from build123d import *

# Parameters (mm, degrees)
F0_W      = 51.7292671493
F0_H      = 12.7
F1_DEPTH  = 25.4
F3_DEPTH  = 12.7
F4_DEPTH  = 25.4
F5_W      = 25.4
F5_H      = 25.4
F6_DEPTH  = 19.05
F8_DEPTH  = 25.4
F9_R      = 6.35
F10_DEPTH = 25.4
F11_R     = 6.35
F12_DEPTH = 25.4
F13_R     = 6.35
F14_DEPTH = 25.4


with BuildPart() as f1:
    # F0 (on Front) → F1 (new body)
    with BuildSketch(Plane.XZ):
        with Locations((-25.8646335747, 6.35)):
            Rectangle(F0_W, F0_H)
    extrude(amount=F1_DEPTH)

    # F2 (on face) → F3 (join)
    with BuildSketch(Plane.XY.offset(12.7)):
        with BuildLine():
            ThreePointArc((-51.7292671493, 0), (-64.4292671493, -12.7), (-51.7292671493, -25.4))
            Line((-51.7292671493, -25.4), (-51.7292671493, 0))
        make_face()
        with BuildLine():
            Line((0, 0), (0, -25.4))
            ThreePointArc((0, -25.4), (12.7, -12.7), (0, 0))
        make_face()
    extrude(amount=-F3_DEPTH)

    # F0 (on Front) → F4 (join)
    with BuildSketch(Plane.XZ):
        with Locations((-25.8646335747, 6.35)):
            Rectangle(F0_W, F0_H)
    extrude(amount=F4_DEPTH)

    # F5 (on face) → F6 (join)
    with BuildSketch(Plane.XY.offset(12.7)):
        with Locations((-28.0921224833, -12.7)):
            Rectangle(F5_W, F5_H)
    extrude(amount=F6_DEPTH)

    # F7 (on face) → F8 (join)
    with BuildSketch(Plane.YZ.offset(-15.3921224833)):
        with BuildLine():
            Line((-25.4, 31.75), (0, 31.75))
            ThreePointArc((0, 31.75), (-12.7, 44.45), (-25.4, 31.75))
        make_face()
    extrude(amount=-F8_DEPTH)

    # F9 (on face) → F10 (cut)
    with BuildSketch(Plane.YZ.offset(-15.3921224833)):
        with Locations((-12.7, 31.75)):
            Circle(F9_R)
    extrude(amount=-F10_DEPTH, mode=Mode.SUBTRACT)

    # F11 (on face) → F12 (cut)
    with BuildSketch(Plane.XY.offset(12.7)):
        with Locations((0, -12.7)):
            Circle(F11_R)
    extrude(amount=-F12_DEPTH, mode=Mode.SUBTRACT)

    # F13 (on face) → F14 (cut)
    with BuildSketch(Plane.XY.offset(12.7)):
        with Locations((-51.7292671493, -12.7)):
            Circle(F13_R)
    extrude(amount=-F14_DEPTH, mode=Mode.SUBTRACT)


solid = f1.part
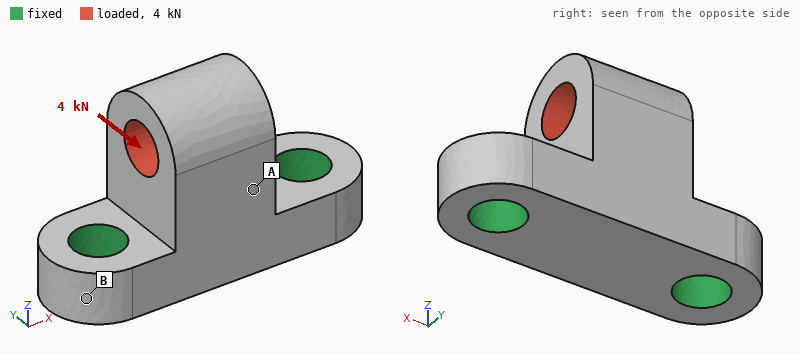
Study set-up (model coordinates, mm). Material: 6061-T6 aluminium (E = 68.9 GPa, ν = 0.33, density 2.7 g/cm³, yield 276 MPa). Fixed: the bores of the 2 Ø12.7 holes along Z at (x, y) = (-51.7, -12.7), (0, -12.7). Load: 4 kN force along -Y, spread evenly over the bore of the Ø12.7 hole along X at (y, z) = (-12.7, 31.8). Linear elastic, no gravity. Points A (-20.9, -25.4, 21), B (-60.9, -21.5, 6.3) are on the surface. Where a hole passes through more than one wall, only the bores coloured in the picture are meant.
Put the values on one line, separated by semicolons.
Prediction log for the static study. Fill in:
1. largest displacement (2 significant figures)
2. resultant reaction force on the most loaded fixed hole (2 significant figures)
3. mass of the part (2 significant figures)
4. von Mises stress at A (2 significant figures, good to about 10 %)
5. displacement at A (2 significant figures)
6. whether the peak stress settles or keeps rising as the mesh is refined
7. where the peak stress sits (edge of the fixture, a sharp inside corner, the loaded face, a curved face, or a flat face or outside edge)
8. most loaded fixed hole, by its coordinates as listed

90 µm; 2.3 kN; 96 g; 22 MPa; 42 µm; keeps rising; edge of the fixture; (-51.7, -12.7)
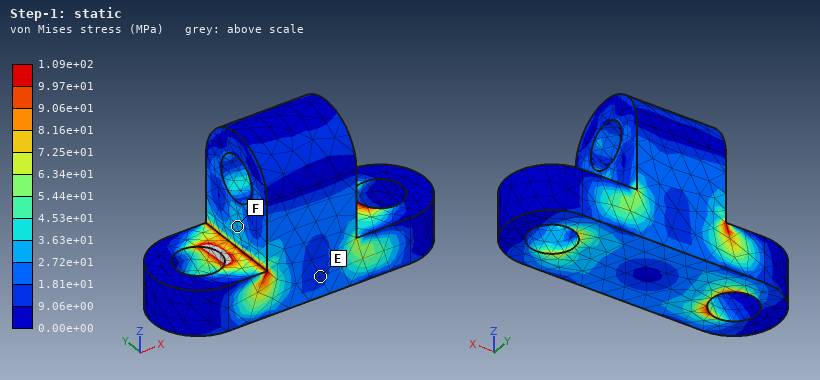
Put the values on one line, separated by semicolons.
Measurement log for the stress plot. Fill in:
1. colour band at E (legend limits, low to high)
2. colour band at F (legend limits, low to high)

9.06e+00 to 1.81e+01 MPa; 2.72e+01 to 3.63e+01 MPa
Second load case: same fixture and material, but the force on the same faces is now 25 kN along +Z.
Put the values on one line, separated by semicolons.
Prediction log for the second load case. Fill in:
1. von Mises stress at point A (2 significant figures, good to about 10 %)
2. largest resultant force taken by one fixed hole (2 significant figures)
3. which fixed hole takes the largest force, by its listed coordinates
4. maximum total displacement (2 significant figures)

52 MPa; 14 kN; (-51.7, -12.7); 64 µm
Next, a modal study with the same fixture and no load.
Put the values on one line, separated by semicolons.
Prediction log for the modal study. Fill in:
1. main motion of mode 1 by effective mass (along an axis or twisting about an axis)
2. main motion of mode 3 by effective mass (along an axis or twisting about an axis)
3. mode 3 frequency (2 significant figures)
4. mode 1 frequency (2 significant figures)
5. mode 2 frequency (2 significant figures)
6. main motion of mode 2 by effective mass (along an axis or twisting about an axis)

along Y; along Z; 17 kHz; 6900 Hz; 12 kHz; along X
